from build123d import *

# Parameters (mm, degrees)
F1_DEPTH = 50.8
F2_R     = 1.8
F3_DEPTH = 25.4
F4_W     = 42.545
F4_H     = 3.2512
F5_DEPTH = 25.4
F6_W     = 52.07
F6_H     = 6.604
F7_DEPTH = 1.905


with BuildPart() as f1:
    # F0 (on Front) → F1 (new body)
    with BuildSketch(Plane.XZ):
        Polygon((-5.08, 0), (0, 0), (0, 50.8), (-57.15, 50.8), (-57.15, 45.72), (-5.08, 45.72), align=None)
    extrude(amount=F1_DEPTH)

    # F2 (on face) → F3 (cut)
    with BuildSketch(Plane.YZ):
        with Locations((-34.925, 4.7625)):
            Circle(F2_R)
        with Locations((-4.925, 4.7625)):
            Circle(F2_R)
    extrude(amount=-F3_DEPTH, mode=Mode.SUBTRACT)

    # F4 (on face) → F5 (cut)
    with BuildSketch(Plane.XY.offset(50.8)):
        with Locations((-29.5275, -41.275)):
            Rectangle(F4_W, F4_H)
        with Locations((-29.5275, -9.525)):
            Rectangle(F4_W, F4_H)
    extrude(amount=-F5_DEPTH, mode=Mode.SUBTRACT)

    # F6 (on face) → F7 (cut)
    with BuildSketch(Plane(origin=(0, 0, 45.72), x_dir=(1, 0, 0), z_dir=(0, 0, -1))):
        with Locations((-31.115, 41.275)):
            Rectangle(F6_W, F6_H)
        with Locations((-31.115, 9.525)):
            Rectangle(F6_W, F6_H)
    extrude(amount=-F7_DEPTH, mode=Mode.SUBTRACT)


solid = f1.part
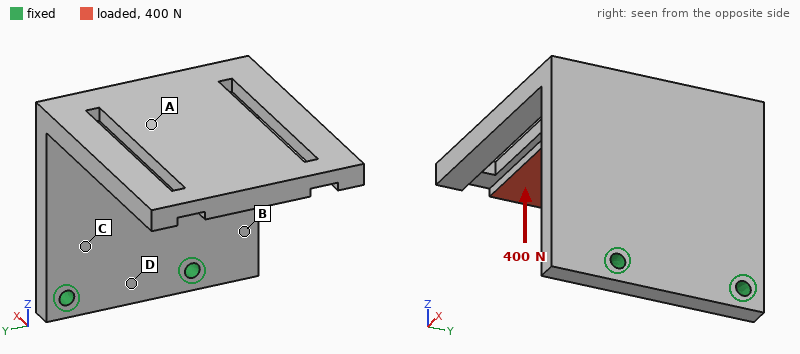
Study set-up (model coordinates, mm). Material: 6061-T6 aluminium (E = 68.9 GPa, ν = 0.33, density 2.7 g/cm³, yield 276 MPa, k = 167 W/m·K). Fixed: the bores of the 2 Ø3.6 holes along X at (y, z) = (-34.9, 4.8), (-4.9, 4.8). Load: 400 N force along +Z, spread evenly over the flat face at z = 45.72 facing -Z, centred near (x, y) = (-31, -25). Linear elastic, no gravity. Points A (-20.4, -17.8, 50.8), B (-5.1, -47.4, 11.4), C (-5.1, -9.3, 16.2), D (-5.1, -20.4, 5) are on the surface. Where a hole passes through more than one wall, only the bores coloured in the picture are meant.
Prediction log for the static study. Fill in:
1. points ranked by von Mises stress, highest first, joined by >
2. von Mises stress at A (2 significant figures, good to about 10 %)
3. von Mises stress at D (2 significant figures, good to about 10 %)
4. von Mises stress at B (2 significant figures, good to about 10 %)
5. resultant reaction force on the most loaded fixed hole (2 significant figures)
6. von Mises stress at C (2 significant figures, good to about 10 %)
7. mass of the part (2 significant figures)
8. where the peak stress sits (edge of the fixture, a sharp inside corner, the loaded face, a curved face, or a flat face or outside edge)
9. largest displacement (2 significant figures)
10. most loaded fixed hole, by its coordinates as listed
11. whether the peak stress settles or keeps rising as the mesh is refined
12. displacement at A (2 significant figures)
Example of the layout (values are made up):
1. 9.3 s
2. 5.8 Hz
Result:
1. C > B > A > D
2. 27 MPa
3. 15 MPa
4. 42 MPa
5. 270 N
6. 52 MPa
7. 65 g
8. edge of the fixture
9. 1.0 mm
10. (-34.9, 4.8)
11. keeps rising
12. 0.45 mm
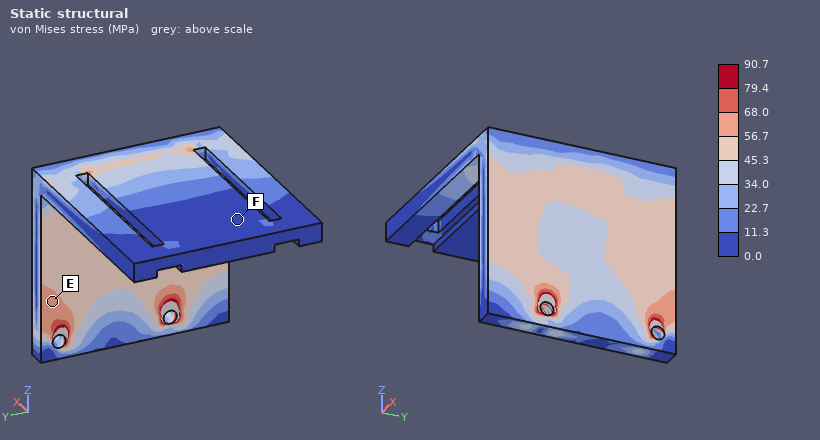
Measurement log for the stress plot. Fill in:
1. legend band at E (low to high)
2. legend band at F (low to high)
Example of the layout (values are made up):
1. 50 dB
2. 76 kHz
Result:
1. 56.7 to 68.0 MPa
2. 0.0 to 11.3 MPa
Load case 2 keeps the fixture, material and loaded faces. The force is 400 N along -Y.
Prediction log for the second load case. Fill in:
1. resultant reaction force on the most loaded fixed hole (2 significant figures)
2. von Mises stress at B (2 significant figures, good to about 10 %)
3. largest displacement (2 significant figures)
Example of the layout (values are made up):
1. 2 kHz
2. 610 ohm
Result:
1. 650 N
2. 23 MPa
3. 0.41 mm
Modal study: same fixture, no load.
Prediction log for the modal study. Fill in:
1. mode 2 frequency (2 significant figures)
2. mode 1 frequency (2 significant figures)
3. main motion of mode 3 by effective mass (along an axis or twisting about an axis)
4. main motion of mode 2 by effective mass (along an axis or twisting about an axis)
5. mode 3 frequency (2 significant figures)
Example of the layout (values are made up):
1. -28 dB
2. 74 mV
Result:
1. 1000 Hz
2. 590 Hz
3. along X
4. along Y
5. 1600 Hz
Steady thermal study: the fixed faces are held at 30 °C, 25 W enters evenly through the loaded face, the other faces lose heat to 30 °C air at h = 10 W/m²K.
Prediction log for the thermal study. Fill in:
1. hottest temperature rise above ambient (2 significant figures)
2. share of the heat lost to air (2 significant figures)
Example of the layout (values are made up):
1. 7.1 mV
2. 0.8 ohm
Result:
1. 45 K
2. 10 %
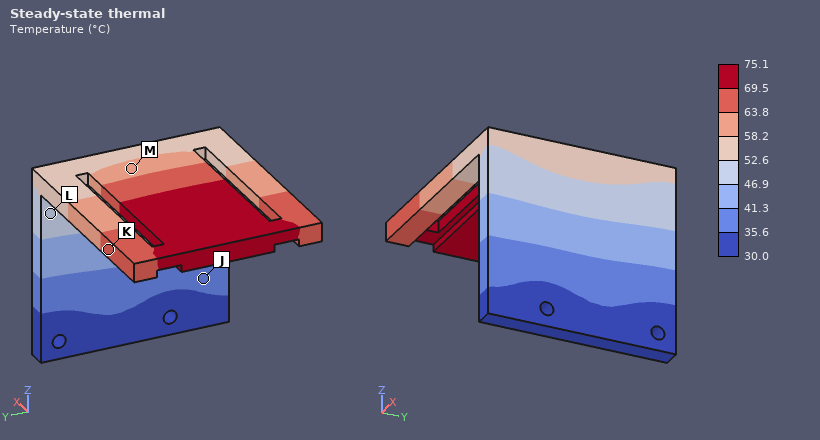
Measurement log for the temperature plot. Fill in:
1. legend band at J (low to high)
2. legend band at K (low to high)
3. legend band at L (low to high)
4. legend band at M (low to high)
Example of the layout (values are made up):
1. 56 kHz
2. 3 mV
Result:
1. 35.6 to 41.3 °C
2. 63.8 to 69.5 °C
3. 46.9 to 52.6 °C
4. 58.2 to 63.8 °C
